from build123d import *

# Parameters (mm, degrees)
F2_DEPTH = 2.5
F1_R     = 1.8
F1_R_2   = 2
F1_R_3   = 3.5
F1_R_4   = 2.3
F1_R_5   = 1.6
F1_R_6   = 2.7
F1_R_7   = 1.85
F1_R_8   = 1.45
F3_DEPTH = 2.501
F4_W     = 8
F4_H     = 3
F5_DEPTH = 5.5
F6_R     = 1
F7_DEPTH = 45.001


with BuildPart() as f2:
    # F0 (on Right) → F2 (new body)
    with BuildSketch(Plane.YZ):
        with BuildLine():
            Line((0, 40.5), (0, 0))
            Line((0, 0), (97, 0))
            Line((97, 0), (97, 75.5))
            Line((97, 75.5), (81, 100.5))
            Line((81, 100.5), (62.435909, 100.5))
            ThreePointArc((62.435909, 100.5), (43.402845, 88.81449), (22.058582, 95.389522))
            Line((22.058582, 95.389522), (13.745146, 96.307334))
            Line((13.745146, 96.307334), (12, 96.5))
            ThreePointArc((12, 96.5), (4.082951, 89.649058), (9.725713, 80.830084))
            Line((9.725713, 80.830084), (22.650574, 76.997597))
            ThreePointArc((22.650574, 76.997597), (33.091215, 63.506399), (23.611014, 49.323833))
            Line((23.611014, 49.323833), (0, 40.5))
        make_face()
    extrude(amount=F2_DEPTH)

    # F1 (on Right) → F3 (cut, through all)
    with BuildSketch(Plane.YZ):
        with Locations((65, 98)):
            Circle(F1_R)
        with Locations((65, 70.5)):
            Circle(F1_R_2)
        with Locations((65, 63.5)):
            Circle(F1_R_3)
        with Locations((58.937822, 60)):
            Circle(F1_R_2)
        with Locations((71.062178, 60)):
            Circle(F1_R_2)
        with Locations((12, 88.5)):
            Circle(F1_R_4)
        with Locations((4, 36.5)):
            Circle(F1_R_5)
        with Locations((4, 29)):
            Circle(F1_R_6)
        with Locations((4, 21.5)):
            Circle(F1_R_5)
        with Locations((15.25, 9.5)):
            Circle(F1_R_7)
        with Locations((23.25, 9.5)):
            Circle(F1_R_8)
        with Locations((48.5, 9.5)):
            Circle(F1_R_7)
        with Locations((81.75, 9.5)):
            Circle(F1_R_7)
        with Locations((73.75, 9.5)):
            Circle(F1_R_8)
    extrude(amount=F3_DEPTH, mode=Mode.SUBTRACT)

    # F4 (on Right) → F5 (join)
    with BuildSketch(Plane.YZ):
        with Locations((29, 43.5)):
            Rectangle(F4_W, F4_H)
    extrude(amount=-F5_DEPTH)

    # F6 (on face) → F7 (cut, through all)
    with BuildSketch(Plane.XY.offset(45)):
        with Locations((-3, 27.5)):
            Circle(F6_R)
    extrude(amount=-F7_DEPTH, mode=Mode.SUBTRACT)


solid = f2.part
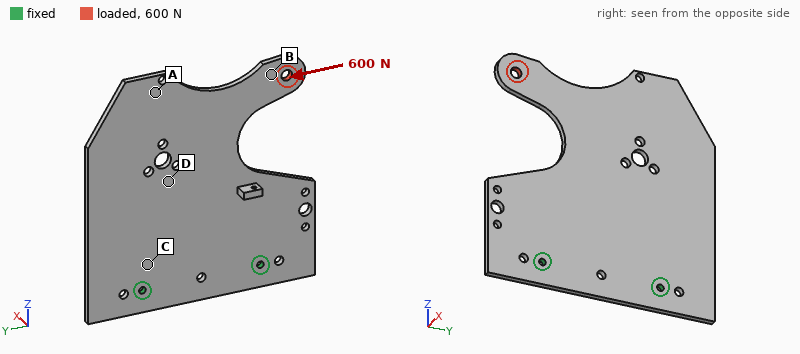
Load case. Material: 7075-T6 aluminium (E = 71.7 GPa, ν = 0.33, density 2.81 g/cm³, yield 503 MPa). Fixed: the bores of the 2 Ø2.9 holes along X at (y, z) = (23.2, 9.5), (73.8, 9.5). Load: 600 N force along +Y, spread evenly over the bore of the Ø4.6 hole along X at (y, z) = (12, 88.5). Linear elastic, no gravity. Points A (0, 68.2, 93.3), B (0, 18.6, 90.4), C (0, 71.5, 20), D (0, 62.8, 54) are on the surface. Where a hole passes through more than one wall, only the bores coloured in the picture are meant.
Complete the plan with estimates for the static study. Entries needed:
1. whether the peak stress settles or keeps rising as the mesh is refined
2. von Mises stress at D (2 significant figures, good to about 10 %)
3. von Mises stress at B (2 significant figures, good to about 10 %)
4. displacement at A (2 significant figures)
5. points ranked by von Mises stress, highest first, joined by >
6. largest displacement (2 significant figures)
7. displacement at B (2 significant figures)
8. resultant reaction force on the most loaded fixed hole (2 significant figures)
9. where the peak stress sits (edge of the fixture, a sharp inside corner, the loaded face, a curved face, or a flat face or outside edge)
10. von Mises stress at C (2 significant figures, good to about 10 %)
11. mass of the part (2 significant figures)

keeps rising
11 MPa
23 MPa
42 µm
B > C > D > A
95 µm
73 µm
1000 N
edge of the fixture
16 MPa
55 g
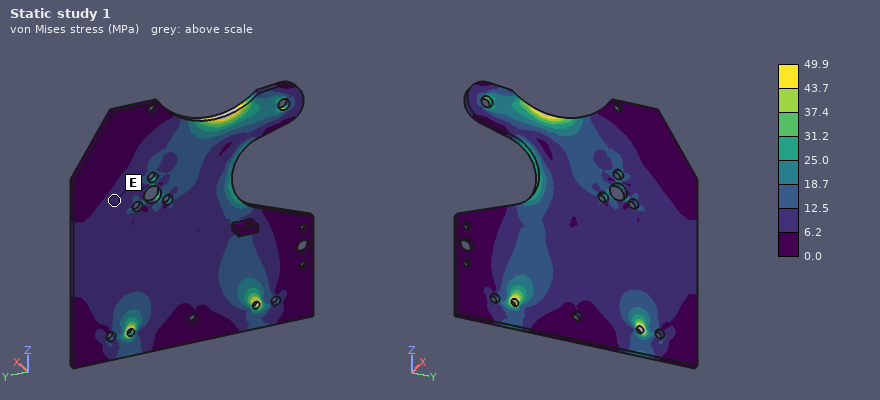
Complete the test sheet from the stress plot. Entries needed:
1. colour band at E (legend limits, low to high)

6.2 to 12.5 MPa
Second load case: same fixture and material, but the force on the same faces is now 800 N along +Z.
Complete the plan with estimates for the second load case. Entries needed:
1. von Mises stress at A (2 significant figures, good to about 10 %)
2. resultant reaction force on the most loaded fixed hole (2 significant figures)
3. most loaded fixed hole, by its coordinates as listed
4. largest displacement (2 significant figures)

6.9 MPa
990 N
(23.2, 9.5)
0.21 mm
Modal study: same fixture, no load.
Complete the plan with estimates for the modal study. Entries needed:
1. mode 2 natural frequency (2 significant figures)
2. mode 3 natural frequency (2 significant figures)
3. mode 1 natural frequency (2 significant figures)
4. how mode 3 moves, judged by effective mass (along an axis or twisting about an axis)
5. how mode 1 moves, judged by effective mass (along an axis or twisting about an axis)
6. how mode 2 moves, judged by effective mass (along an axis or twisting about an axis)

630 Hz
1500 Hz
270 Hz
along X
along X
twisting about Z
